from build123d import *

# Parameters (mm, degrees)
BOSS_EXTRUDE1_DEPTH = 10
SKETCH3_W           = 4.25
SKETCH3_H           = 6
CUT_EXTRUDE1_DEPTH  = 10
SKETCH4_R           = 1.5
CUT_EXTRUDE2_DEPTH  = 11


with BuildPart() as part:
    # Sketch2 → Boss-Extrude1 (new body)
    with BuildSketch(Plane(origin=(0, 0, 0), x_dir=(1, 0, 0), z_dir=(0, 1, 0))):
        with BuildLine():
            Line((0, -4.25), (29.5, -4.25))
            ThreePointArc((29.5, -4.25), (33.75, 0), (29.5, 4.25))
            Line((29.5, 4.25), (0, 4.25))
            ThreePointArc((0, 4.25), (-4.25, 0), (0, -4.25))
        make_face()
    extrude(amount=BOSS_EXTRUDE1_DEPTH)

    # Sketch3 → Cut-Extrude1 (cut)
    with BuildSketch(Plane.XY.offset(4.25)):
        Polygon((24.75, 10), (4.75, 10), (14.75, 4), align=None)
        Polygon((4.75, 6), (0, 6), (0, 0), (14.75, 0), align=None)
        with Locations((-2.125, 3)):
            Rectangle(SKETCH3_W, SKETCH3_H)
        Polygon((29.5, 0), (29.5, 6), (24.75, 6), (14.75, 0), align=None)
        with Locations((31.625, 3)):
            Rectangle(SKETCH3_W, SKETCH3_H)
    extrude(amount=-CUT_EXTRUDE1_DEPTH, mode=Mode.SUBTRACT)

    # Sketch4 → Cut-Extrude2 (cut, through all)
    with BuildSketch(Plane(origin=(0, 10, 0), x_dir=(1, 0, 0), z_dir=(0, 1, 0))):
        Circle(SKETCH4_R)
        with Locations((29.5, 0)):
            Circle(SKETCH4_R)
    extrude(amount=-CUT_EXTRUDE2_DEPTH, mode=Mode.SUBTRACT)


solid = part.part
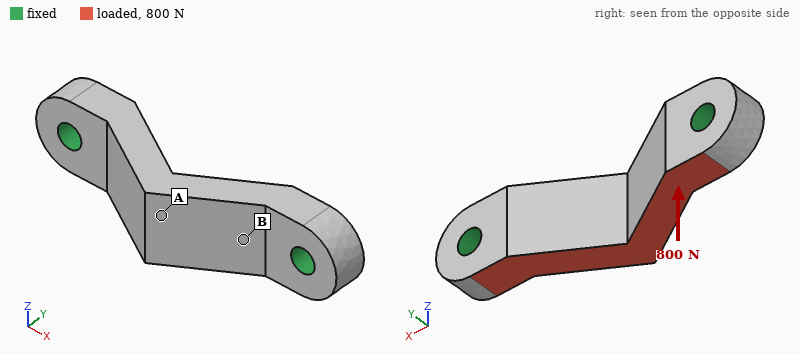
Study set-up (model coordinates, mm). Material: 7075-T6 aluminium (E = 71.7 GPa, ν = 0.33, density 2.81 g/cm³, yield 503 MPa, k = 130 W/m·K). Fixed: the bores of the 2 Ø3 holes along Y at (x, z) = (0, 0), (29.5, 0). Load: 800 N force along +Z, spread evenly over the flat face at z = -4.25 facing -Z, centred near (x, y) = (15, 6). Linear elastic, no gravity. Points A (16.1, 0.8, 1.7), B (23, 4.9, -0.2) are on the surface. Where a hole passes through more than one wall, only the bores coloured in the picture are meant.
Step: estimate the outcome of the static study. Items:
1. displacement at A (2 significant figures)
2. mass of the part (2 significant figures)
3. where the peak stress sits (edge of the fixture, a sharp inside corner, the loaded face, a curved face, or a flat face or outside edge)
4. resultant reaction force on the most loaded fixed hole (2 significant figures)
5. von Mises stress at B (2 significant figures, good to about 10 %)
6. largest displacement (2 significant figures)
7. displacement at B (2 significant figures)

25 µm
3.3 g
edge of the fixture
400 N
45 MPa
29 µm
11 µm
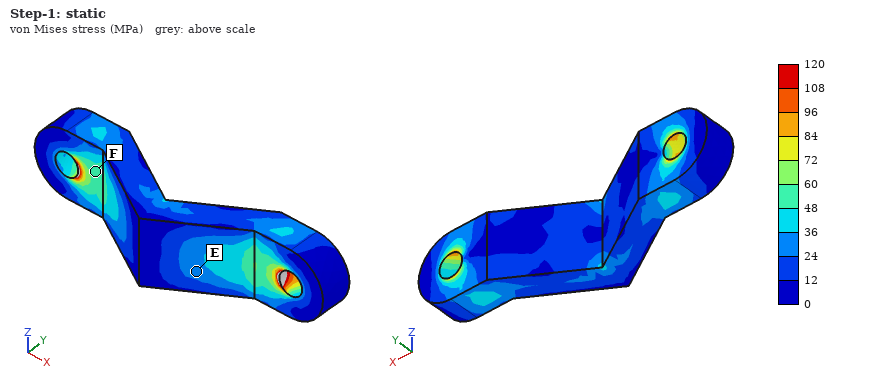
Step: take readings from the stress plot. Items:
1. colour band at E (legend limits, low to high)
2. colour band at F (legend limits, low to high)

24 to 36 MPa
48 to 60 MPa
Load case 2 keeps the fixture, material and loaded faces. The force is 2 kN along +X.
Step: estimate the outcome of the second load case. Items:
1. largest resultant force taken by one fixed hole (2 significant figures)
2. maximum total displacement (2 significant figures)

1.0 kN
11 µm
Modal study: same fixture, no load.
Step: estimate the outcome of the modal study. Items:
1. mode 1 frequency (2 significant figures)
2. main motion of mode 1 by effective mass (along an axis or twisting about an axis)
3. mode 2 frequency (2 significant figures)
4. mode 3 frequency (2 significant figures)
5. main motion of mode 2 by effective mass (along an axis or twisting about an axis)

20 kHz
along Z
32 kHz
47 kHz
along Y
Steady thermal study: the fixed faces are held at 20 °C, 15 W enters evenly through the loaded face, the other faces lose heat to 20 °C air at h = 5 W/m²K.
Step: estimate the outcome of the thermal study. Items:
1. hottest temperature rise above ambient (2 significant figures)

17 K
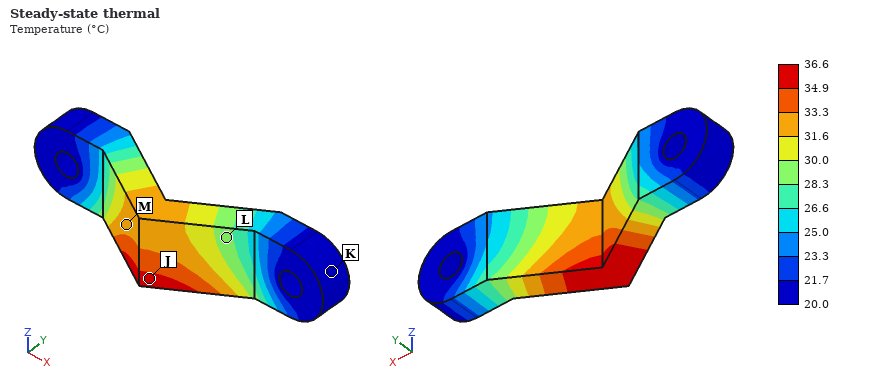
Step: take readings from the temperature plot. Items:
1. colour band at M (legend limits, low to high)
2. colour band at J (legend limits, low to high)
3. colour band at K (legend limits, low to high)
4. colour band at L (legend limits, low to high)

31.6 to 33.3 °C
34.9 to 36.6 °C
20.0 to 21.7 °C
28.3 to 30.0 °C
